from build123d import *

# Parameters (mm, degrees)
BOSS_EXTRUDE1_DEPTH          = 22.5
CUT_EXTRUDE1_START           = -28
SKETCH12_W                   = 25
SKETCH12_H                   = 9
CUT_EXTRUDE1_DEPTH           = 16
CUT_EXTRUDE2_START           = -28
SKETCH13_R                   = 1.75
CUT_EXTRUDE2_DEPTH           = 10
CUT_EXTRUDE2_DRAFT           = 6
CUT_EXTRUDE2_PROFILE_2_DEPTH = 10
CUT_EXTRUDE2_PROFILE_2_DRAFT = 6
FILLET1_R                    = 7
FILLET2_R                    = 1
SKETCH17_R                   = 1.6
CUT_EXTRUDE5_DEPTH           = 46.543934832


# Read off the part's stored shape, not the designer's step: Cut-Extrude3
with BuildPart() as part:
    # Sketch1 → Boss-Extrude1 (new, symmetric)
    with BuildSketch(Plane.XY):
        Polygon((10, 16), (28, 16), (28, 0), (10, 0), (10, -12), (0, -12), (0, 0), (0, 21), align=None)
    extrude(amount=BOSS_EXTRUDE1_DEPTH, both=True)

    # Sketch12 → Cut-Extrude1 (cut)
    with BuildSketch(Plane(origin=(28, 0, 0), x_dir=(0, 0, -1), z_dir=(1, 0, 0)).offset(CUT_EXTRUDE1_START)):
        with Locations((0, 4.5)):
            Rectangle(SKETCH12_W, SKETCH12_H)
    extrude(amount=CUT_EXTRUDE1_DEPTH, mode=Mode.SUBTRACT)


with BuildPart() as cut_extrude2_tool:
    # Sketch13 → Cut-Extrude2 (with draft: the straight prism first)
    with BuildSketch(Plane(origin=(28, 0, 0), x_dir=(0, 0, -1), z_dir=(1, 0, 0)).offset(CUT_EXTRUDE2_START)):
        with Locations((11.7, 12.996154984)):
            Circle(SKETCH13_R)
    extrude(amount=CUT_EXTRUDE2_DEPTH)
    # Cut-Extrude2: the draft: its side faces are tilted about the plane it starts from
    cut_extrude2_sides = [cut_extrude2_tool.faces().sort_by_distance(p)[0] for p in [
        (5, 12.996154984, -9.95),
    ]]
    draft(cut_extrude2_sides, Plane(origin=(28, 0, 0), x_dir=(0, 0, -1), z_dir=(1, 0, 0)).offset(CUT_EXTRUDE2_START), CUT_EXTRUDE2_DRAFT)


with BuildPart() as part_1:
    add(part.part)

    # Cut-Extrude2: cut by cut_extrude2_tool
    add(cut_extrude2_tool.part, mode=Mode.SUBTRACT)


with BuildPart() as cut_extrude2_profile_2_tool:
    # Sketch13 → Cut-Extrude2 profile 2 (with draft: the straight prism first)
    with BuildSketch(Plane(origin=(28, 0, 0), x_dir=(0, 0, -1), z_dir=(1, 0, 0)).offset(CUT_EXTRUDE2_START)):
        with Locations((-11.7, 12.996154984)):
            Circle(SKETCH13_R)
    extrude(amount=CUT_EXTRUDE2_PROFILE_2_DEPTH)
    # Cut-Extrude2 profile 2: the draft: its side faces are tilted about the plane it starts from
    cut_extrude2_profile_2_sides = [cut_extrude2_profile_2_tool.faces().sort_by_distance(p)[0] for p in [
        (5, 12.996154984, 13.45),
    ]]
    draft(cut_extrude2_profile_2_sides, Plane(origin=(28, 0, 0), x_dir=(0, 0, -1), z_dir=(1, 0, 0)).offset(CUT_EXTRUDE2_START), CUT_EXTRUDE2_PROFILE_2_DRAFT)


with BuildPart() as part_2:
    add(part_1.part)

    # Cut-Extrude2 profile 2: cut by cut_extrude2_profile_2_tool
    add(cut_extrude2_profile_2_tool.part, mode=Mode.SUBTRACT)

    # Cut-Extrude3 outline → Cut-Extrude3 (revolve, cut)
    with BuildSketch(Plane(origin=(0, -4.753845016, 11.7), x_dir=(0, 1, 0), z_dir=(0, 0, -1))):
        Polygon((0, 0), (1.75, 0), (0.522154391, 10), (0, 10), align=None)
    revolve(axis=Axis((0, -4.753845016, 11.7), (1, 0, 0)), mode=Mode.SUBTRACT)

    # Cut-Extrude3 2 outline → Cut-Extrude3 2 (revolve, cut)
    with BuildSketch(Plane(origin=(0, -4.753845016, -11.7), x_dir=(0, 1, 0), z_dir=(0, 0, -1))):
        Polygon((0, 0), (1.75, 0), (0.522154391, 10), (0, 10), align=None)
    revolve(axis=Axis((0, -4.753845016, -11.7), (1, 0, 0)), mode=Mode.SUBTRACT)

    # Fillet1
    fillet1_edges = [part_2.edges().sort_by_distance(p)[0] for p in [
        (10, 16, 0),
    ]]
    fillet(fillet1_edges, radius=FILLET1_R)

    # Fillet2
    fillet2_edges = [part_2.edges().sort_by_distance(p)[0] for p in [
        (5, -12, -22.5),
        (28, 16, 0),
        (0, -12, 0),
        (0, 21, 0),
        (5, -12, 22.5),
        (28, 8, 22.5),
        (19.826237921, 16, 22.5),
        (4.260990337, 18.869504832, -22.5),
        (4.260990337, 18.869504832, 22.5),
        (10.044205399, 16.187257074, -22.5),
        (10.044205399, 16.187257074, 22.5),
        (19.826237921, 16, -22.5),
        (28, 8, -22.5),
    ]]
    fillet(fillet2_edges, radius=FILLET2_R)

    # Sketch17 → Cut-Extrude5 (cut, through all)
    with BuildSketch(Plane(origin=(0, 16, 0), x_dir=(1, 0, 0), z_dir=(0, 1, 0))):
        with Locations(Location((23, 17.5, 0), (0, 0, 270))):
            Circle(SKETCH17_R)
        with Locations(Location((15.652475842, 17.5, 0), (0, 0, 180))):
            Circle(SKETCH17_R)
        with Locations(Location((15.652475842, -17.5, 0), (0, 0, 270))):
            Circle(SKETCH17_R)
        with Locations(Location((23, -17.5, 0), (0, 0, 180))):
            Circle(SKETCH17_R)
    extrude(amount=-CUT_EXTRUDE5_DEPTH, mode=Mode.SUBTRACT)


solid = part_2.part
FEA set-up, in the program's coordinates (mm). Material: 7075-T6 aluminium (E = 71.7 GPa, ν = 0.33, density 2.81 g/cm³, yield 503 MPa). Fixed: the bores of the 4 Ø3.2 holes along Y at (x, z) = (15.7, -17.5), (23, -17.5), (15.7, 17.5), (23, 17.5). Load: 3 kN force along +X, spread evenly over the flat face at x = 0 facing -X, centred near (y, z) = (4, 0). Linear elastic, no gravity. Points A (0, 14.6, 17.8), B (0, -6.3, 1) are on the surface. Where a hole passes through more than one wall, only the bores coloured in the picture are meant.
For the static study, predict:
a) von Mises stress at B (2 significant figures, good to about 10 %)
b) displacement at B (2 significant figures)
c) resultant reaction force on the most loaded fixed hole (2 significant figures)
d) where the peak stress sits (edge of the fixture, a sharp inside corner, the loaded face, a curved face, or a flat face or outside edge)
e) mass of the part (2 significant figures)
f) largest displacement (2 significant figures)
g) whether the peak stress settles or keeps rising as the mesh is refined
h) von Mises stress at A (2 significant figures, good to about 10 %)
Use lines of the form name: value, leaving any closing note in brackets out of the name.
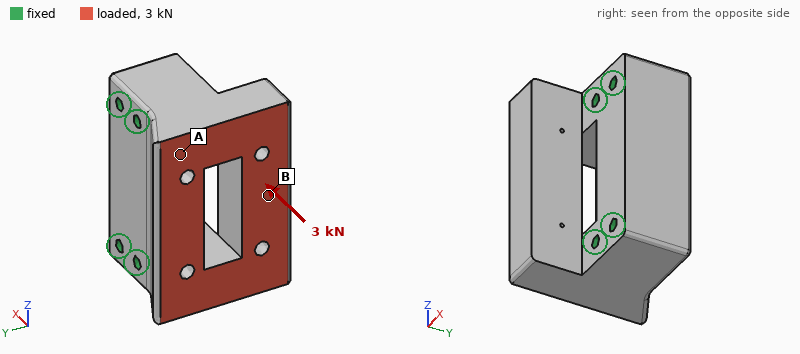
von Mises stress at B: 11 MPa
displacement at B: 15 µm
resultant reaction force on the most loaded fixed hole: 1.2 kN
where the peak stress sits: a sharp inside corner
mass of the part: 63 g
largest displacement: 19 µm
whether the peak stress settles or keeps rising as the mesh is refined: keeps rising
von Mises stress at A: 4.5 MPa
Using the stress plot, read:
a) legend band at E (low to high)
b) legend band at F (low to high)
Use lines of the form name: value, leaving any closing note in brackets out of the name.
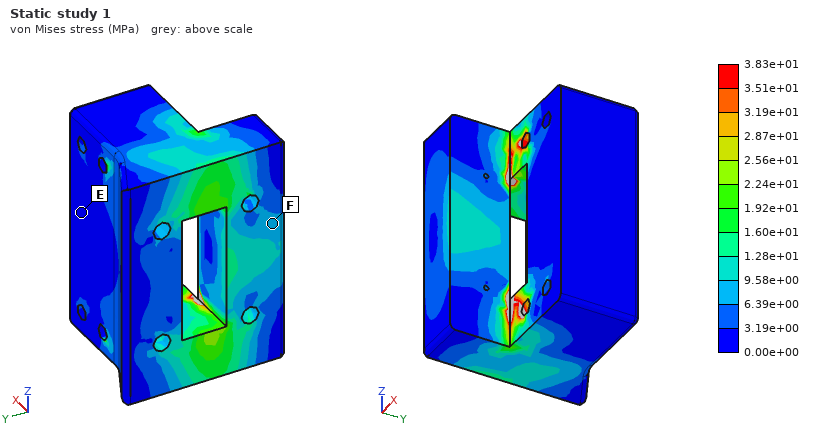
legend band at E: 0.00e+00 to 3.19e+00 MPa
legend band at F: 6.39e+00 to 9.58e+00 MPa
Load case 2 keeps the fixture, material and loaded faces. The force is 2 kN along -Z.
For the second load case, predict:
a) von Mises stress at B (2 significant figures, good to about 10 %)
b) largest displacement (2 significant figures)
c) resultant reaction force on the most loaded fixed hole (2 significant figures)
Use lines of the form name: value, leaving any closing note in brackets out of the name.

von Mises stress at B: 6.4 MPa
largest displacement: 8.7 µm
resultant reaction force on the most loaded fixed hole: 1.2 kN
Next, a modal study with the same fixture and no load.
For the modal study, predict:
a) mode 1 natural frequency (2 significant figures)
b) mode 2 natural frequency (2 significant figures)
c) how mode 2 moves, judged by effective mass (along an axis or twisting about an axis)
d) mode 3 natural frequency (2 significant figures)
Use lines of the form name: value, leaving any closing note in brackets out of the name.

mode 1 natural frequency: 12 kHz
mode 2 natural frequency: 16 kHz
how mode 2 moves, judged by effective mass: along Z
mode 3 natural frequency: 21 kHz
